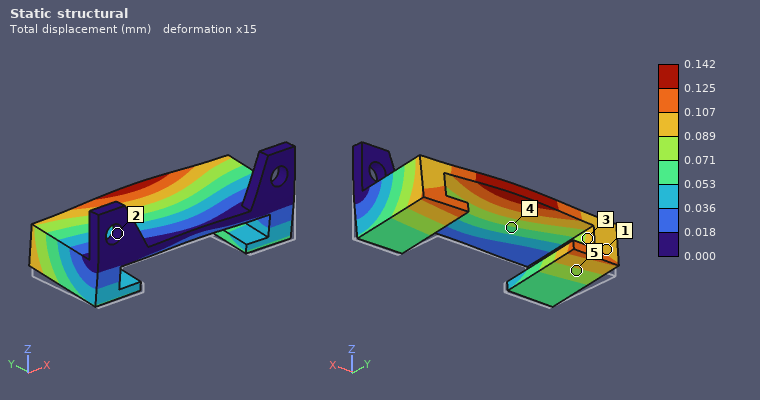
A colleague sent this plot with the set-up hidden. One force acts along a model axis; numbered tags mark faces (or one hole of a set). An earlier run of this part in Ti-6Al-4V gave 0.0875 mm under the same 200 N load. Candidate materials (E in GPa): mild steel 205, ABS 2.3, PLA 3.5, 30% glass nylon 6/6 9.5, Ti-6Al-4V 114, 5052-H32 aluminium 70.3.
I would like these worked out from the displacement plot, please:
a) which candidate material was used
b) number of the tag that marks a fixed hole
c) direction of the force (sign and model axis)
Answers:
5052-H32 aluminium
2
+Z
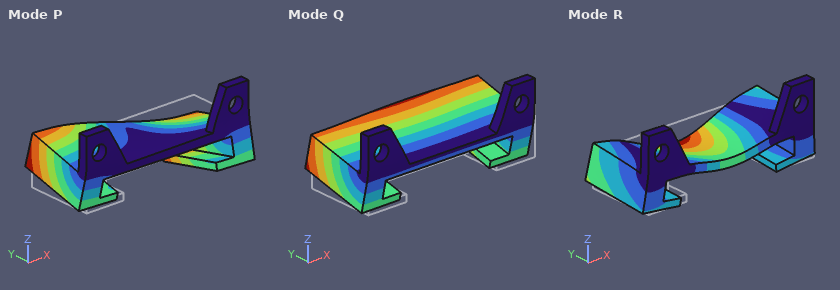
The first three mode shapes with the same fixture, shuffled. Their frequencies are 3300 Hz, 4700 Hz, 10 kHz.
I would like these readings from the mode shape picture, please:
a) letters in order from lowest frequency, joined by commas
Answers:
Q, P, R
